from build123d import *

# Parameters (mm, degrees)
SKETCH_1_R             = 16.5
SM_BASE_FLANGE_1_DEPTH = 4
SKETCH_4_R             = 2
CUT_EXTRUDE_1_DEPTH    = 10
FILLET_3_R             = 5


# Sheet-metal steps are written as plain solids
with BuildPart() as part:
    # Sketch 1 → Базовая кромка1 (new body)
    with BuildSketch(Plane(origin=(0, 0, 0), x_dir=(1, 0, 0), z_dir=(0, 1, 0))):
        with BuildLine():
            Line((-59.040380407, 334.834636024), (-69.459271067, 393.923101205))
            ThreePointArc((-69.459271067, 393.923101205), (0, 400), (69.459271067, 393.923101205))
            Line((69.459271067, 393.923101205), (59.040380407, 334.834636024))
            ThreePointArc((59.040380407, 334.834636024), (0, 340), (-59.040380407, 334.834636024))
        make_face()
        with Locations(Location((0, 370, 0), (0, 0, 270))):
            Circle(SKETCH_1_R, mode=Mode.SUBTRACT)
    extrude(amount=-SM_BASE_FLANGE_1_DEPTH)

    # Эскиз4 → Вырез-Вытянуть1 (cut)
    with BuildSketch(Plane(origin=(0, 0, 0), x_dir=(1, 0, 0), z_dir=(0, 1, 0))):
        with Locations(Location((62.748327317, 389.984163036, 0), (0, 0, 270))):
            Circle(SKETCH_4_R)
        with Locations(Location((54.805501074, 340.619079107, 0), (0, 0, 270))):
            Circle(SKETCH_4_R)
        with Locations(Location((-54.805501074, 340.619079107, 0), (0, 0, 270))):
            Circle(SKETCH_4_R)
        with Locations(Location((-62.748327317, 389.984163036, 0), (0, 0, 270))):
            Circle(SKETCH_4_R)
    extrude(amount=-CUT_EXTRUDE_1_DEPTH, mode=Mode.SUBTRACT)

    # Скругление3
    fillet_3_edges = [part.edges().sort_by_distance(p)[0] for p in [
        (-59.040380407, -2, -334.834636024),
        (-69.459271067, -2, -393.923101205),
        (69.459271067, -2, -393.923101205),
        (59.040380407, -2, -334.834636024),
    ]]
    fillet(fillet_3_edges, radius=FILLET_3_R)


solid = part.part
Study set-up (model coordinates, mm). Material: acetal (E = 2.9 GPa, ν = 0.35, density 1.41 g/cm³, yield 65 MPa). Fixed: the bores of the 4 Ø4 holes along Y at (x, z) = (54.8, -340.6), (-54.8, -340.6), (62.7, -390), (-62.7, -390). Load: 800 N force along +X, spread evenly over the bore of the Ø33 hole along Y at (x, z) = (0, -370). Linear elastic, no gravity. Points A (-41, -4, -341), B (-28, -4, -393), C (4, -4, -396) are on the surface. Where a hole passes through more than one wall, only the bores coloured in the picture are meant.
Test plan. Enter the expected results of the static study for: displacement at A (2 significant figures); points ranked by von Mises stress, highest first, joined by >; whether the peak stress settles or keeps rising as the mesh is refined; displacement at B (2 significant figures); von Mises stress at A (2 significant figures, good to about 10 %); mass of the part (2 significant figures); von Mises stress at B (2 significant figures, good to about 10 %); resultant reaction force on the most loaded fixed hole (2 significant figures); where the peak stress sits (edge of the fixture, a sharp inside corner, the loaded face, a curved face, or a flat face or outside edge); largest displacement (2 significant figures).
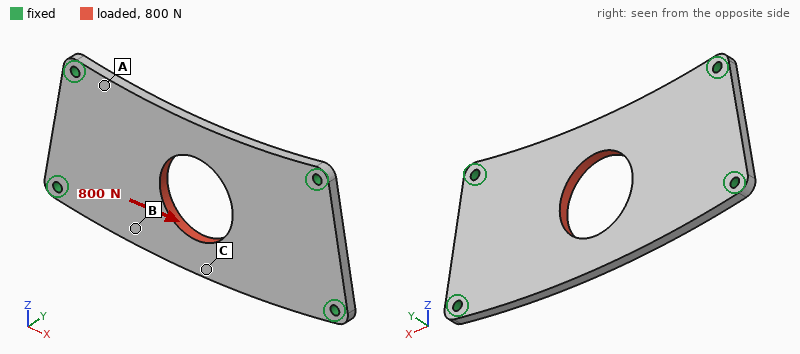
14 µm
A > B > C
keeps rising
34 µm
2.7 MPa
38 g
1.6 MPa
230 N
edge of the fixture
53 µm
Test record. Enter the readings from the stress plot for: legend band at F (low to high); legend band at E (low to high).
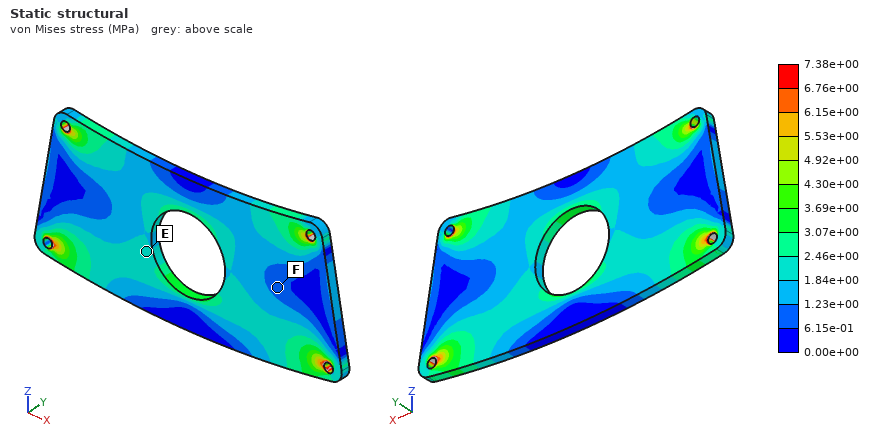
6.15e-01 to 1.23e+00 MPa
1.84e+00 to 2.46e+00 MPa
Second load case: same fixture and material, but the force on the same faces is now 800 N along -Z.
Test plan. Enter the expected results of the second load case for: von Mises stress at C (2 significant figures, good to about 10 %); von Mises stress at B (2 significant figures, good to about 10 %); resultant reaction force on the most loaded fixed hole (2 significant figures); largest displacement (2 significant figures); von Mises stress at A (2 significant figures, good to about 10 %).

4.5 MPa
1.6 MPa
340 N
0.14 mm
3.3 MPa
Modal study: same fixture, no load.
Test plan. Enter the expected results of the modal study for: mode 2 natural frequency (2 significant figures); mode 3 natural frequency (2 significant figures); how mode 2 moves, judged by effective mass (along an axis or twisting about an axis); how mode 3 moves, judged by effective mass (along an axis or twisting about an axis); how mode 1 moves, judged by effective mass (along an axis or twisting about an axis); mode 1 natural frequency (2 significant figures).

690 Hz
950 Hz
twisting about X
twisting about Z
along Y
380 Hz
